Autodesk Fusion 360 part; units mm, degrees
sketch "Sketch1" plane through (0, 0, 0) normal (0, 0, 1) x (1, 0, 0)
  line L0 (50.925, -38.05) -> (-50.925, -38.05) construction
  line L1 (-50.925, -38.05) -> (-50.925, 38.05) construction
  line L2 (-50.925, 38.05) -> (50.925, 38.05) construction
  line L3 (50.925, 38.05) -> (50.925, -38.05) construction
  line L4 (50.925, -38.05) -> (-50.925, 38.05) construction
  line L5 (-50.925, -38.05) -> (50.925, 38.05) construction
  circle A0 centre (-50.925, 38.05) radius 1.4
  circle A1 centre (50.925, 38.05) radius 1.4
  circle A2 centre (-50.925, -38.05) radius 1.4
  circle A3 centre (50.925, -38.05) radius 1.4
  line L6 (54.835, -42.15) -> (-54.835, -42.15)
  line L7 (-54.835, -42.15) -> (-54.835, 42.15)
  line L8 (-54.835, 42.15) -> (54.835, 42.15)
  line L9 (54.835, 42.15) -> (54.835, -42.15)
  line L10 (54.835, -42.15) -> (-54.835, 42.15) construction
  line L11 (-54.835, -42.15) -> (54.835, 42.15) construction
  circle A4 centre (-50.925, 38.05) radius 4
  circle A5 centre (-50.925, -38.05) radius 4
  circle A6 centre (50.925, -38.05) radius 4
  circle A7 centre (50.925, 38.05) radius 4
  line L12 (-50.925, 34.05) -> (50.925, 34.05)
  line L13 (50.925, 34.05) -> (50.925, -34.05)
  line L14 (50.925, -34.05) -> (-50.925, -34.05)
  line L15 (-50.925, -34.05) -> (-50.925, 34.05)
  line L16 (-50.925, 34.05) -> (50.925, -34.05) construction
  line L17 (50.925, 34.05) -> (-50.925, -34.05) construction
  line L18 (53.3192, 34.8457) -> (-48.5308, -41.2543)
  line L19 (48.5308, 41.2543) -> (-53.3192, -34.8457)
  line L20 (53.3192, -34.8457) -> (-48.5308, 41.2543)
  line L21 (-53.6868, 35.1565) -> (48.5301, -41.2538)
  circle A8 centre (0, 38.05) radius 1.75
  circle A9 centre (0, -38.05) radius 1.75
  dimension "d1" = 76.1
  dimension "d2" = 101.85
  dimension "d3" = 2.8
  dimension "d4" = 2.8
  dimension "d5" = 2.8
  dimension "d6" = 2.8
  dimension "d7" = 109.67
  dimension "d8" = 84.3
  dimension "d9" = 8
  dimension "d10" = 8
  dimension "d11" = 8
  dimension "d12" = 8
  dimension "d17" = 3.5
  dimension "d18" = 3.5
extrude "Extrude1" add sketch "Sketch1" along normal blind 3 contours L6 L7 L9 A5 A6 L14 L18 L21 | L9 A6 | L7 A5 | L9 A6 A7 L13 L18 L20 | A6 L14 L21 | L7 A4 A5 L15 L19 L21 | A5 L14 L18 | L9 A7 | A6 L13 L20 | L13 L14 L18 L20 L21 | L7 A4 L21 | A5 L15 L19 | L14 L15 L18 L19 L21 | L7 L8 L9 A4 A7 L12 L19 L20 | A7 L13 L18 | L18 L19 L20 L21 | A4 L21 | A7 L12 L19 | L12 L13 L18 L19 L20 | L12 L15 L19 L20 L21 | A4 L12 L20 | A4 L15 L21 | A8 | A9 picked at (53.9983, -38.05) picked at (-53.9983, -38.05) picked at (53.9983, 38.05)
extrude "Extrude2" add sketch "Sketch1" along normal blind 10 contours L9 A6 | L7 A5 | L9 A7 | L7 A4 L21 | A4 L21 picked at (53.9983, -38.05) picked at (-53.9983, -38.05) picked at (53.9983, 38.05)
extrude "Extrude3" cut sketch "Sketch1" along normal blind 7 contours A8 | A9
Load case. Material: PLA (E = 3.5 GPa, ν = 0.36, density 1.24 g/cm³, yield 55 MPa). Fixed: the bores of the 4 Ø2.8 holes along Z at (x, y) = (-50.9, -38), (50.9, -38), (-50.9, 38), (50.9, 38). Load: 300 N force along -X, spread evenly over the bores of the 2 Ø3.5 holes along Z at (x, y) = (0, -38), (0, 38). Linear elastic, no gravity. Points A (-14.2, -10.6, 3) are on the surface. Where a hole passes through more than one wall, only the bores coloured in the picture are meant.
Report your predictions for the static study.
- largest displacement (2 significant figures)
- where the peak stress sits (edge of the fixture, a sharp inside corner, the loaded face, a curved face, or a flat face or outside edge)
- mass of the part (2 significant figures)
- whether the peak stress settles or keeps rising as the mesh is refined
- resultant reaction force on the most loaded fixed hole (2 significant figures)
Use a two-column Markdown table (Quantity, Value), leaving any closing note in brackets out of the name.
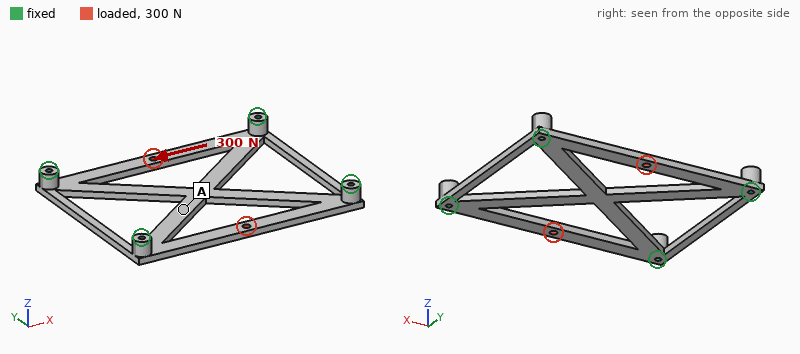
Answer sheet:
| Quantity | Value |
|---|---|
| largest displacement | 45 µm |
| where the peak stress sits | edge of the fixture |
| mass of the part | 16 g |
| whether the peak stress settles or keeps rising as the mesh is refined | keeps rising |
| resultant reaction force on the most loaded fixed hole | 75 N |
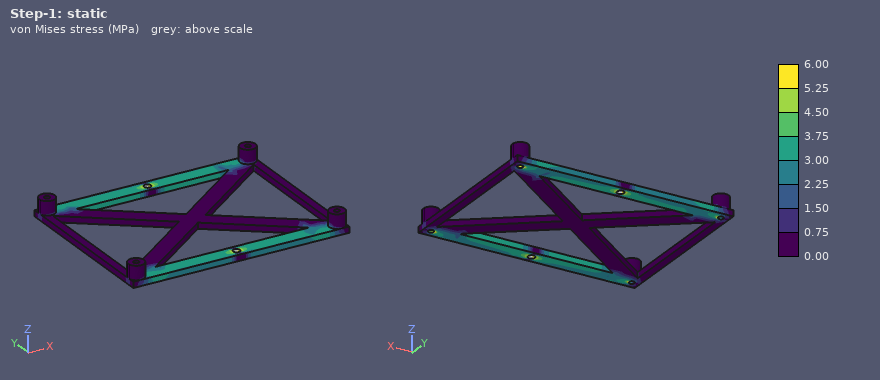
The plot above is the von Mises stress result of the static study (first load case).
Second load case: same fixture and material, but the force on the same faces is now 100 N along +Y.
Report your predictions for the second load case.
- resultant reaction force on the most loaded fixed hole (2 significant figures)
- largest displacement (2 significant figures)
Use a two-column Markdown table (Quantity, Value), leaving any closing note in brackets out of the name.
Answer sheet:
| Quantity | Value |
|---|---|
| resultant reaction force on the most loaded fixed hole | 25 N |
| largest displacement | 0.52 mm |
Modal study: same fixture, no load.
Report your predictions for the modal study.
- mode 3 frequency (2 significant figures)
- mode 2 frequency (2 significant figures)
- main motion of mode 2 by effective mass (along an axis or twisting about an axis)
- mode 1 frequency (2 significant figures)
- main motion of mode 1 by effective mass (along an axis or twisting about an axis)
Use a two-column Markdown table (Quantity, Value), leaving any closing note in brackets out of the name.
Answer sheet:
| Quantity | Value |
|---|---|
| mode 3 frequency | 610 Hz |
| mode 2 frequency | 580 Hz |
| main motion of mode 2 by effective mass | twisting about X |
| mode 1 frequency | 390 Hz |
| main motion of mode 1 by effective mass | along Z |
